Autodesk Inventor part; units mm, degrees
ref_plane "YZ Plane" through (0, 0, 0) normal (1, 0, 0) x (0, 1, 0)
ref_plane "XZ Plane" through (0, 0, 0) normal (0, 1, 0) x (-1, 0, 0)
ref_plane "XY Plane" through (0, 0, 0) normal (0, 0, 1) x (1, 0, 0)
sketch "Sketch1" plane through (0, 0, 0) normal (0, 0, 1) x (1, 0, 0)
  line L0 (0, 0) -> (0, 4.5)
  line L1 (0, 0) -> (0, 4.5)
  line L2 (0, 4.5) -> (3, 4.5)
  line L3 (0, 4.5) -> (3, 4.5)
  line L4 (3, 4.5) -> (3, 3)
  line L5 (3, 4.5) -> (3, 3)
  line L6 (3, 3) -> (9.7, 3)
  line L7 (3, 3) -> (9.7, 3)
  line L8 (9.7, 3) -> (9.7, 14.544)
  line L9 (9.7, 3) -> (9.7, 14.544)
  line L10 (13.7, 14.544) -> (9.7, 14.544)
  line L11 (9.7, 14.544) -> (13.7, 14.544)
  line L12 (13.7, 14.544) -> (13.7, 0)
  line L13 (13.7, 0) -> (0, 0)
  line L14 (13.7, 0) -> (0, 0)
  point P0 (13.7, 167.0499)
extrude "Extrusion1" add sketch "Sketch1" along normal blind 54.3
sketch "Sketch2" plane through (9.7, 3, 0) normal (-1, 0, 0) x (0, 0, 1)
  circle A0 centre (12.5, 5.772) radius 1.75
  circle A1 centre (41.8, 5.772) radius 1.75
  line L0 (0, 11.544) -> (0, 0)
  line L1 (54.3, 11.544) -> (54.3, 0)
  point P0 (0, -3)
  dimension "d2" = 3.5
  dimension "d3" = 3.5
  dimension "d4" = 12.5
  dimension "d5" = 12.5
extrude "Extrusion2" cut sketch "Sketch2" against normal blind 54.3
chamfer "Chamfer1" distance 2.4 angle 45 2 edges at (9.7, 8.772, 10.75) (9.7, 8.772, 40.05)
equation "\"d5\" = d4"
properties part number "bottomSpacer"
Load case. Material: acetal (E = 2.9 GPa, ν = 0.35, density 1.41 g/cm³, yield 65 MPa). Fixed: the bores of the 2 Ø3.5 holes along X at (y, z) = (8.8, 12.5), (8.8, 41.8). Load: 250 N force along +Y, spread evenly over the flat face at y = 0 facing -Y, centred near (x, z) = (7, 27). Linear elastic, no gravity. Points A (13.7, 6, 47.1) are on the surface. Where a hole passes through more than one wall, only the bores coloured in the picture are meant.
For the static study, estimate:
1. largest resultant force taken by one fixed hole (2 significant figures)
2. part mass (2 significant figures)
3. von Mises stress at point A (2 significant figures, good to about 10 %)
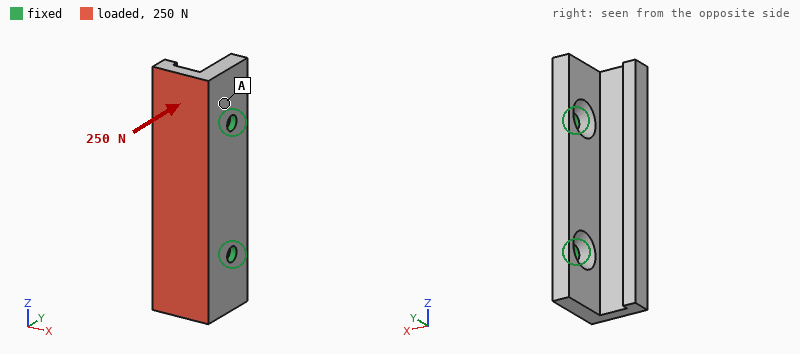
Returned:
130 N
6.8 g
9.1 MPa
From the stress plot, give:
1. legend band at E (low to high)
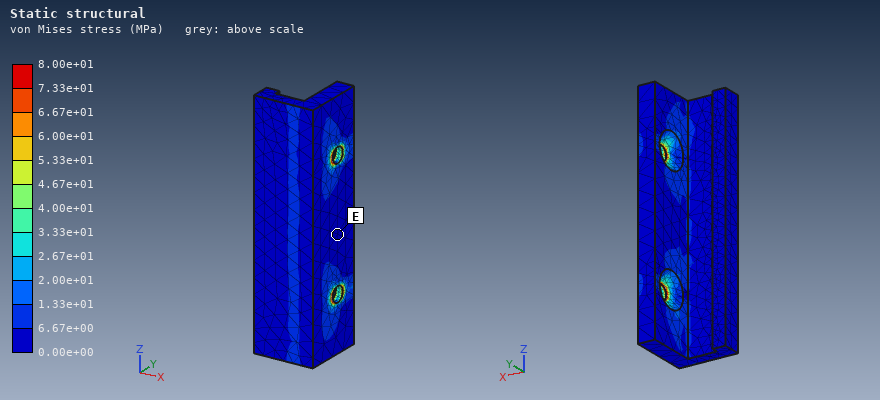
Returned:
0.00e+00 to 6.67e+00 MPa
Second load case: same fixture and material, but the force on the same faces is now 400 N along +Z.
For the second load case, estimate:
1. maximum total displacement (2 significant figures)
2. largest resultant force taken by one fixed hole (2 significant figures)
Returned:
0.14 mm
240 N
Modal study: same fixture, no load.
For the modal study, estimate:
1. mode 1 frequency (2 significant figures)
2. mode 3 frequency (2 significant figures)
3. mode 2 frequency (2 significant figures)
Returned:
1700 Hz
4500 Hz
2400 Hz
